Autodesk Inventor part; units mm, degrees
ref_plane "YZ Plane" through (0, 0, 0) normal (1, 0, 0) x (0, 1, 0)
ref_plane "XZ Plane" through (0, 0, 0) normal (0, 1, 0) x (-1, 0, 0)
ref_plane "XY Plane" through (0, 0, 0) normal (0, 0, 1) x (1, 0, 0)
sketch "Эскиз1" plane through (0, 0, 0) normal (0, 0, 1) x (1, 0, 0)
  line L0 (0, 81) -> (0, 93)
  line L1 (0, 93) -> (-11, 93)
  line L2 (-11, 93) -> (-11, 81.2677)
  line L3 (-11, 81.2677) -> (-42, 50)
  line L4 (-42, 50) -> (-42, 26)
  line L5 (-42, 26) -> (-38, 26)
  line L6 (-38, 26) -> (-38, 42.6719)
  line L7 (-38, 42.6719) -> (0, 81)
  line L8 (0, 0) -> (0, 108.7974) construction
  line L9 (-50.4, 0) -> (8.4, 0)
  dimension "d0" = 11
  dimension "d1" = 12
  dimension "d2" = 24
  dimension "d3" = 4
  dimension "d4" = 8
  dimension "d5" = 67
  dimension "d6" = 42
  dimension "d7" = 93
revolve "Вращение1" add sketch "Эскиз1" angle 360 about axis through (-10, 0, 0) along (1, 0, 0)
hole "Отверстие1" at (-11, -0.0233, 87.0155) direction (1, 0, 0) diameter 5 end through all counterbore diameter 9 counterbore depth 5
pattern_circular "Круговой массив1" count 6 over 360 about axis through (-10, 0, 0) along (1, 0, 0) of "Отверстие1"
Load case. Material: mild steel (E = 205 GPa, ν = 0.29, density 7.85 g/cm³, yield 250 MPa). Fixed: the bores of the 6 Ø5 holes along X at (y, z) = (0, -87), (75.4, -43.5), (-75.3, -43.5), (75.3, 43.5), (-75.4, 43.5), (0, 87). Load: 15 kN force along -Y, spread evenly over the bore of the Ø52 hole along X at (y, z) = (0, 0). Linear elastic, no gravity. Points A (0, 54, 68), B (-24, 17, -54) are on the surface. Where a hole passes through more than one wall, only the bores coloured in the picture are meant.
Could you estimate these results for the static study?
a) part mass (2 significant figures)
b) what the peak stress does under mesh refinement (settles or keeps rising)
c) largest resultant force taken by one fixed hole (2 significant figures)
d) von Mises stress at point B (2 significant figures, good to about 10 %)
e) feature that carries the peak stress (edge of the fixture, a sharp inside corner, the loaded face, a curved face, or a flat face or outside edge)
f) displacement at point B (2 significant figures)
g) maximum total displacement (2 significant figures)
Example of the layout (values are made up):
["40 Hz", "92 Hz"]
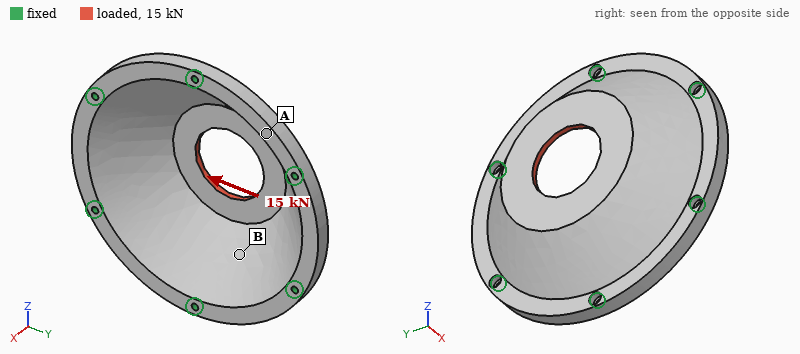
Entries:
["1.9 kg", "keeps rising", "3.1 kN", "19 MPa", "edge of the fixture", "4.2 µm", "22 µm"]
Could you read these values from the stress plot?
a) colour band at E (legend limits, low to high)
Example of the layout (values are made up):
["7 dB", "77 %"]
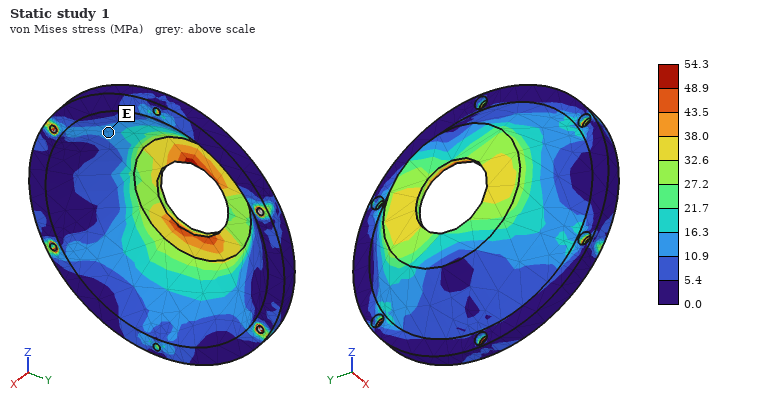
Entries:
["10.9 to 16.3 MPa"]
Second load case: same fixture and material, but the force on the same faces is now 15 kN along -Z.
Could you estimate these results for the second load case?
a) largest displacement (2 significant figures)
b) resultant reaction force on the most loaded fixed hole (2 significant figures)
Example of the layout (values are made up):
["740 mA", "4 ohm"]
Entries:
["22 µm", "3.3 kN"]
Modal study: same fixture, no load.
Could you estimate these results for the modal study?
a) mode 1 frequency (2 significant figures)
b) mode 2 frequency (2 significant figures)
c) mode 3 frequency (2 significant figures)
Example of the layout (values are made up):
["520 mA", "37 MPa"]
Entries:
["6200 Hz", "6300 Hz", "6300 Hz"]
